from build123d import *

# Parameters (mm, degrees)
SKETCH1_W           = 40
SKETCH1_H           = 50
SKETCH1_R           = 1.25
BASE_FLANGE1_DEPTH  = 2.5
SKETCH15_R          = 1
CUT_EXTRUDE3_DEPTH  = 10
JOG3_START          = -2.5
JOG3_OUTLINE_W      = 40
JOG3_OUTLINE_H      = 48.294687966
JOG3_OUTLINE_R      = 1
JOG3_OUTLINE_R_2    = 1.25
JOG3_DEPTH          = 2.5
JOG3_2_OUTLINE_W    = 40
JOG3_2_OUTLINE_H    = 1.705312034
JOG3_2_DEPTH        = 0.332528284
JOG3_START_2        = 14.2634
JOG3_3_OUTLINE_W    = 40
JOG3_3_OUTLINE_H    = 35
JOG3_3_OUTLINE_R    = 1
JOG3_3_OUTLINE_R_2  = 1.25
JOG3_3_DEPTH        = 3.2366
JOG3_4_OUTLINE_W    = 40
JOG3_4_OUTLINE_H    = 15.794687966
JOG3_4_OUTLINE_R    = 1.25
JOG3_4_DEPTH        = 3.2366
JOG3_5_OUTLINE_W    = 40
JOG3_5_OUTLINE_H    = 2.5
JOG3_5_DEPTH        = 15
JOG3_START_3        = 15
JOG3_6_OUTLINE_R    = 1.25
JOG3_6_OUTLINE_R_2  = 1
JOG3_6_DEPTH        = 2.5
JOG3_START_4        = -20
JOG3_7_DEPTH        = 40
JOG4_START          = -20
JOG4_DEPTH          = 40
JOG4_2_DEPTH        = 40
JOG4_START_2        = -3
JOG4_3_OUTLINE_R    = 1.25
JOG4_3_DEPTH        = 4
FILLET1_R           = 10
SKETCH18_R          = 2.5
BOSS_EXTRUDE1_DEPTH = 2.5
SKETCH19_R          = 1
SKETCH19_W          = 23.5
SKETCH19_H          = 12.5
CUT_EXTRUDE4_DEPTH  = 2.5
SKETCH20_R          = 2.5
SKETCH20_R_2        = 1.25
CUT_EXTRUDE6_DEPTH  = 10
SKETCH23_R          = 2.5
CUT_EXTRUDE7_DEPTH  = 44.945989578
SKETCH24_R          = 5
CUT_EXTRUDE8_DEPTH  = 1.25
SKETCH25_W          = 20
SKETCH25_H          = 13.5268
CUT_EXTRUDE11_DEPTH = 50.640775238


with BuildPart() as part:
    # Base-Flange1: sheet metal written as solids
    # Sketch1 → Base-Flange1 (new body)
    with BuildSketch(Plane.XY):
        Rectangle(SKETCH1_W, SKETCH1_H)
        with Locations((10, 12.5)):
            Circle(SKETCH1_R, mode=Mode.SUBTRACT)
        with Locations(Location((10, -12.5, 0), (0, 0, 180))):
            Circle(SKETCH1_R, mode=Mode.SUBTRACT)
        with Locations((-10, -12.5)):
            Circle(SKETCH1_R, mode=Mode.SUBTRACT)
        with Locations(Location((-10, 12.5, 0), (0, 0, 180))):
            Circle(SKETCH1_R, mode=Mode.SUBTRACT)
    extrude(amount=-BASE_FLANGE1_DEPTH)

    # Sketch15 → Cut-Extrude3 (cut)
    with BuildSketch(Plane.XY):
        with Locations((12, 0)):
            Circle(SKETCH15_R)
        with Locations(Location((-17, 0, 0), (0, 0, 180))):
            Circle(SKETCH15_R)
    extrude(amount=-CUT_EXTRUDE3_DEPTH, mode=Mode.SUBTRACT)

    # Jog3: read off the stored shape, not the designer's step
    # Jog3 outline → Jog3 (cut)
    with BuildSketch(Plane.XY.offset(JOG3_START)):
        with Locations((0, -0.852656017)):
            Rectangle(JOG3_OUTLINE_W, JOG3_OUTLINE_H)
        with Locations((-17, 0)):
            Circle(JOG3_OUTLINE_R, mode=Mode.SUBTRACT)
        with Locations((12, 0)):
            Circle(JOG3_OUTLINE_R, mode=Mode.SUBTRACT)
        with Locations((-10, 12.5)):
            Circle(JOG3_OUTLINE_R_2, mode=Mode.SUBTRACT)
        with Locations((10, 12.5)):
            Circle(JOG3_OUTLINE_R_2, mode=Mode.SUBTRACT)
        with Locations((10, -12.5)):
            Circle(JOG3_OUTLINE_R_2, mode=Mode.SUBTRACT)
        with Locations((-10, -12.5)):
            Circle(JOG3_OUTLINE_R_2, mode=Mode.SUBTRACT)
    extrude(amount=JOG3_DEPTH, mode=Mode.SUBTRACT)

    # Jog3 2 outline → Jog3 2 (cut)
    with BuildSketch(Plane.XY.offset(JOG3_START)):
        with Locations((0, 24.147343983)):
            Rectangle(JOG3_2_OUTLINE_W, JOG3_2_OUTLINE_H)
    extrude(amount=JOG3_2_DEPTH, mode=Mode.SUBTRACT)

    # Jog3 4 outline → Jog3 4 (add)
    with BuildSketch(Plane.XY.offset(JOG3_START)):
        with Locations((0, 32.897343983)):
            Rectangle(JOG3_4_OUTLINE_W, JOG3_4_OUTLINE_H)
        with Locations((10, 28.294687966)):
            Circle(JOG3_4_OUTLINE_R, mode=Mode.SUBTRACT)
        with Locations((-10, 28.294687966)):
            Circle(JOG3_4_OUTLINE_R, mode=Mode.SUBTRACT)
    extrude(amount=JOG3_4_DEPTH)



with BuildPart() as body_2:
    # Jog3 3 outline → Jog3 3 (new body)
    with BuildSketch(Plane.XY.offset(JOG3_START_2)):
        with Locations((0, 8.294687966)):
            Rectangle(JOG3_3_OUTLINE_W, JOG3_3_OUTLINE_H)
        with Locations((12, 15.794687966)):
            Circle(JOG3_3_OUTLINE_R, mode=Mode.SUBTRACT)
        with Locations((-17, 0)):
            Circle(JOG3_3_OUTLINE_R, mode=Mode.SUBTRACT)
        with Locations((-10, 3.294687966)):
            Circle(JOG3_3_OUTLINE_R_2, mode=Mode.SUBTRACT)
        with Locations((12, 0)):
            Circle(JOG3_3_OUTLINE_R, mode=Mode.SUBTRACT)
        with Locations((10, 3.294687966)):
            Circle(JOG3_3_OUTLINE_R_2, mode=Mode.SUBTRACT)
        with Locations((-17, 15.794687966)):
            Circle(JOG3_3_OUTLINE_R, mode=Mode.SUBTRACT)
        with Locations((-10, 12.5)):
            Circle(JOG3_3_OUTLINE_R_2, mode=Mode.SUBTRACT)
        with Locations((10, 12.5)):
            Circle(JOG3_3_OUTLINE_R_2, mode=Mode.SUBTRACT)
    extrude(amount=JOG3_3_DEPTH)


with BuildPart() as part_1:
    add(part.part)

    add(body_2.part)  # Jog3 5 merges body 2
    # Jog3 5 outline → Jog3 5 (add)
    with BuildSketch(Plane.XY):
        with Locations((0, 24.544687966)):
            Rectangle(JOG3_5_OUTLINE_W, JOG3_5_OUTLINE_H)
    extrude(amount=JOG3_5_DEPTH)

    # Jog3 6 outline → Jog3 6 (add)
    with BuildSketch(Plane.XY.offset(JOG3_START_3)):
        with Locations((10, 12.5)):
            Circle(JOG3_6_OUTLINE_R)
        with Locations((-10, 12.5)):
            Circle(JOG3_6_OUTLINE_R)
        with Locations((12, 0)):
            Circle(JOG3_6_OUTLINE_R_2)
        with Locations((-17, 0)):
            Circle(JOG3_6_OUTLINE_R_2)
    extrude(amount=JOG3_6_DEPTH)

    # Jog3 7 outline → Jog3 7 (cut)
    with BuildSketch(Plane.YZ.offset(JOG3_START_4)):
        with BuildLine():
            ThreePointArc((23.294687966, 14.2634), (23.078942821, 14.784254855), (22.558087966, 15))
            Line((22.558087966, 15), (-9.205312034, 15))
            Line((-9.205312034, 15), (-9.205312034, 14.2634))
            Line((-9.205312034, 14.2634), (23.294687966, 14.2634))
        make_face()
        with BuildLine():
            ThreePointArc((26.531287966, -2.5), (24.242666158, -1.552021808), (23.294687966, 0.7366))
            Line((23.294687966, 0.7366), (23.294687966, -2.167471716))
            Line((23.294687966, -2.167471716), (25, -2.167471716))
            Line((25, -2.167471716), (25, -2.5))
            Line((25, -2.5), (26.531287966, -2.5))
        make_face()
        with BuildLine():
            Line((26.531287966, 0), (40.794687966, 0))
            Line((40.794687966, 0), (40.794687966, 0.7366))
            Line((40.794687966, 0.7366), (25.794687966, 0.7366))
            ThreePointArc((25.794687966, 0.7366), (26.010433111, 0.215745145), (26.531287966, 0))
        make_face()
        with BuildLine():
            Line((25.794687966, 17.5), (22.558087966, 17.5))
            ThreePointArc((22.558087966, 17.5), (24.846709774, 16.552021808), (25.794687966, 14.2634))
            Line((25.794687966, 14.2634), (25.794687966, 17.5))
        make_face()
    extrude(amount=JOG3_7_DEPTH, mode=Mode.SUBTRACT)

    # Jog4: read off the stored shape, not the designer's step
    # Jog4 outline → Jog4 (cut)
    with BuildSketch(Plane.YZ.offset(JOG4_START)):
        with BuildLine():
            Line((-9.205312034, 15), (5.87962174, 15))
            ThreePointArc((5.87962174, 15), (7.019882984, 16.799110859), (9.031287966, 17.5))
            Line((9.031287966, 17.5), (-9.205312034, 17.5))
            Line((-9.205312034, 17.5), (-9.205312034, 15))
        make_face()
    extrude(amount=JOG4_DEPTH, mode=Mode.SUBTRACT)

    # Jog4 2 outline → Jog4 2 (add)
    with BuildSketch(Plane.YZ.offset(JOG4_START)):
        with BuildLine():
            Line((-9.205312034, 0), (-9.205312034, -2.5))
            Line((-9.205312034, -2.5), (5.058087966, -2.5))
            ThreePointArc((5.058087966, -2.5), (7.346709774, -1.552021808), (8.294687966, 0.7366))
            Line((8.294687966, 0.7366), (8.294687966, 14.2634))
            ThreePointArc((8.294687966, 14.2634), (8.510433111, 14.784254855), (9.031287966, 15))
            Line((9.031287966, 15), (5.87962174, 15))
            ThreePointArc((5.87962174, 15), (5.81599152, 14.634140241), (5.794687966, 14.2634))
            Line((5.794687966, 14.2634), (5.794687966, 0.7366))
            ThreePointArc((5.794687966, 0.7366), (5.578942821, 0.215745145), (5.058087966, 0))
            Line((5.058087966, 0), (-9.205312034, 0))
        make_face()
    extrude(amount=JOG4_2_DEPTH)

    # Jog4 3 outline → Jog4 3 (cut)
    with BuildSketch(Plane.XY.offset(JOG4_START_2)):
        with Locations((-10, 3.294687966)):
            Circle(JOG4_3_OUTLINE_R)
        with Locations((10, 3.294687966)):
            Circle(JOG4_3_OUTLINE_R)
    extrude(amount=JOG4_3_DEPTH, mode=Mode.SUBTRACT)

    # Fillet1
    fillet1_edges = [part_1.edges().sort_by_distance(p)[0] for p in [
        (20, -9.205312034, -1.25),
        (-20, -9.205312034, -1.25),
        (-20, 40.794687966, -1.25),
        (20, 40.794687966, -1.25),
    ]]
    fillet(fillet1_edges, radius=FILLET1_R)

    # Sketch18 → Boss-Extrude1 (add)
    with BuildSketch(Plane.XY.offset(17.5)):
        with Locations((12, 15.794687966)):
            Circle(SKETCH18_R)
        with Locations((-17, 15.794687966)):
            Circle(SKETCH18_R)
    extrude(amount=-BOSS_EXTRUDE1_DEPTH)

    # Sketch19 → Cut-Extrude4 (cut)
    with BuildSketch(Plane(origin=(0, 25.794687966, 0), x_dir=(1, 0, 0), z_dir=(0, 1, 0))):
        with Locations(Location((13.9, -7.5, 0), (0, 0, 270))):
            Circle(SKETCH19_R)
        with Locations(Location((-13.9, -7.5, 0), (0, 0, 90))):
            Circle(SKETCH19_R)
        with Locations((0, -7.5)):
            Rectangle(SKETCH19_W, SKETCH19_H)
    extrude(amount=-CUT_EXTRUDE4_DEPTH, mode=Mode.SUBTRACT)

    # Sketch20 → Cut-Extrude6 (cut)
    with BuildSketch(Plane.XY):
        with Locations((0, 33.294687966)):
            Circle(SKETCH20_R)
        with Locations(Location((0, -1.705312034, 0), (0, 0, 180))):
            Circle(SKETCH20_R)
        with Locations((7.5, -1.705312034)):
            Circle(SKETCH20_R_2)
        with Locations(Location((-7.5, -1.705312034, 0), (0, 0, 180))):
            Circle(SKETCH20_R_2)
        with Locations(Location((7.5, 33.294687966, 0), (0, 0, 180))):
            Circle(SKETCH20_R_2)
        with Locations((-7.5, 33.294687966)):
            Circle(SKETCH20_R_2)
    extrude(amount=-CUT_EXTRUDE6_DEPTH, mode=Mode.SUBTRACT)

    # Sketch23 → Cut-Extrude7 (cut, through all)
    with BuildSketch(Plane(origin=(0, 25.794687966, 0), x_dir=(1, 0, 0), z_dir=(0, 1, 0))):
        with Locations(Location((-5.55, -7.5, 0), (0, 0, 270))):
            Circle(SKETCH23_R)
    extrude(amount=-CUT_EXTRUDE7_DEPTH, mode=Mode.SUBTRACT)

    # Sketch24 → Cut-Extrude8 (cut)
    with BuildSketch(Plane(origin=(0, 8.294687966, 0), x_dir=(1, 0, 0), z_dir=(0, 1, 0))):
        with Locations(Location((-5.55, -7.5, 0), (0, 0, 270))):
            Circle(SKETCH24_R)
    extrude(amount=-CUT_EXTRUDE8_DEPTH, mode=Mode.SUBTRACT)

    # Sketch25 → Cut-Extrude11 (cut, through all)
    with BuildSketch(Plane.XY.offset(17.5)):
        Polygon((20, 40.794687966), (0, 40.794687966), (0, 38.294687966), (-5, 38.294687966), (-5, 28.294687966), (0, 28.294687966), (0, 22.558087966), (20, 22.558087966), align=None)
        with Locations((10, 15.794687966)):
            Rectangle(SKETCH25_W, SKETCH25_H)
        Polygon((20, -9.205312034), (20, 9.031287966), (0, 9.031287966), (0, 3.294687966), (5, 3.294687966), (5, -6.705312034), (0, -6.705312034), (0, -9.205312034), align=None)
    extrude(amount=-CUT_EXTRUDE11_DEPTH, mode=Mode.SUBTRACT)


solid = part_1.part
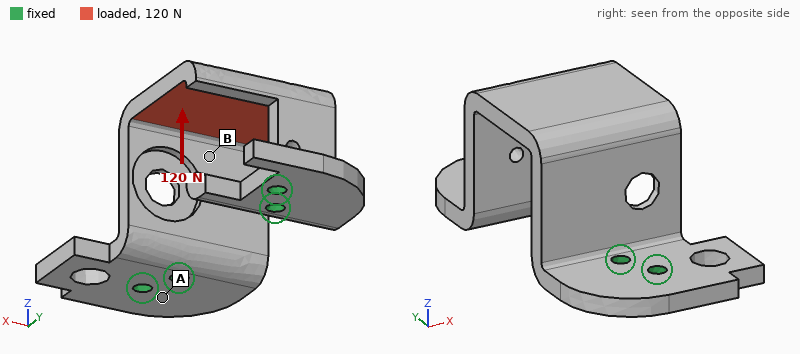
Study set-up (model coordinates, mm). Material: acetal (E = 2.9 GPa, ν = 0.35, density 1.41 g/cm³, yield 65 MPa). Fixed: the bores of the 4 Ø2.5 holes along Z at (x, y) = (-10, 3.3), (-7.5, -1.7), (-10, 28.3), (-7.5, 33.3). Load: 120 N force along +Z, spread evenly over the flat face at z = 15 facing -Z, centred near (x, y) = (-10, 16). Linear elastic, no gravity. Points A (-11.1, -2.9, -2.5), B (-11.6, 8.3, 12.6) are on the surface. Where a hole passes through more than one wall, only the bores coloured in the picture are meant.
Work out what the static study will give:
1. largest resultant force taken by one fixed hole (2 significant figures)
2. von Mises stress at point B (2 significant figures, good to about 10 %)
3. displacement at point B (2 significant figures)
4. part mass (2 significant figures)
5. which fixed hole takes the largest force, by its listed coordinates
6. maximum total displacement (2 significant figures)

66 N
7.7 MPa
0.094 mm
4.8 g
(-10, 28.3)
0.40 mm
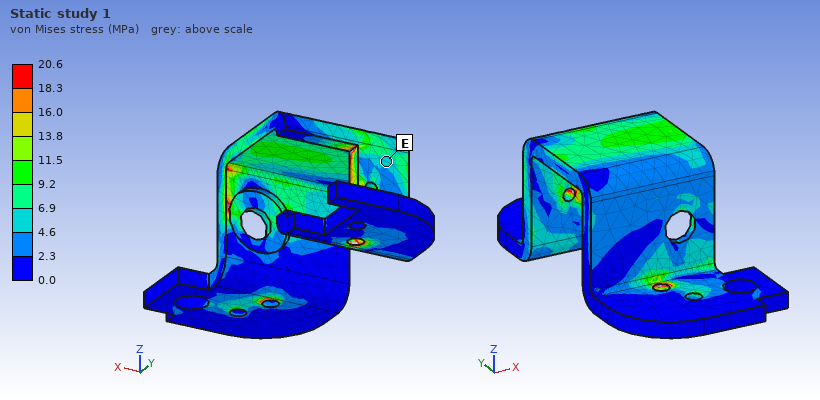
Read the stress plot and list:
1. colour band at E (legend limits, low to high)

4.6 to 6.9 MPa
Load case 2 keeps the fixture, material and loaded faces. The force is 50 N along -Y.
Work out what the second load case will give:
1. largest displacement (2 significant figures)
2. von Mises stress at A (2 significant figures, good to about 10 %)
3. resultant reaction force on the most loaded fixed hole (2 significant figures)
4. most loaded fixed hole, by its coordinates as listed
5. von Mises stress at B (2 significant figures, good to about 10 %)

0.48 mm
3.1 MPa
31 N
(-10, 28.3)
9.5 MPa
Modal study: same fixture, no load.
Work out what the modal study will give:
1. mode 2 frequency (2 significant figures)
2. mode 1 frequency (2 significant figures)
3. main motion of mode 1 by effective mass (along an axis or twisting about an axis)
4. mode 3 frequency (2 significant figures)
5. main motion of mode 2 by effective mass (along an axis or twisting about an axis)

1300 Hz
1200 Hz
along X
2100 Hz
along Y
